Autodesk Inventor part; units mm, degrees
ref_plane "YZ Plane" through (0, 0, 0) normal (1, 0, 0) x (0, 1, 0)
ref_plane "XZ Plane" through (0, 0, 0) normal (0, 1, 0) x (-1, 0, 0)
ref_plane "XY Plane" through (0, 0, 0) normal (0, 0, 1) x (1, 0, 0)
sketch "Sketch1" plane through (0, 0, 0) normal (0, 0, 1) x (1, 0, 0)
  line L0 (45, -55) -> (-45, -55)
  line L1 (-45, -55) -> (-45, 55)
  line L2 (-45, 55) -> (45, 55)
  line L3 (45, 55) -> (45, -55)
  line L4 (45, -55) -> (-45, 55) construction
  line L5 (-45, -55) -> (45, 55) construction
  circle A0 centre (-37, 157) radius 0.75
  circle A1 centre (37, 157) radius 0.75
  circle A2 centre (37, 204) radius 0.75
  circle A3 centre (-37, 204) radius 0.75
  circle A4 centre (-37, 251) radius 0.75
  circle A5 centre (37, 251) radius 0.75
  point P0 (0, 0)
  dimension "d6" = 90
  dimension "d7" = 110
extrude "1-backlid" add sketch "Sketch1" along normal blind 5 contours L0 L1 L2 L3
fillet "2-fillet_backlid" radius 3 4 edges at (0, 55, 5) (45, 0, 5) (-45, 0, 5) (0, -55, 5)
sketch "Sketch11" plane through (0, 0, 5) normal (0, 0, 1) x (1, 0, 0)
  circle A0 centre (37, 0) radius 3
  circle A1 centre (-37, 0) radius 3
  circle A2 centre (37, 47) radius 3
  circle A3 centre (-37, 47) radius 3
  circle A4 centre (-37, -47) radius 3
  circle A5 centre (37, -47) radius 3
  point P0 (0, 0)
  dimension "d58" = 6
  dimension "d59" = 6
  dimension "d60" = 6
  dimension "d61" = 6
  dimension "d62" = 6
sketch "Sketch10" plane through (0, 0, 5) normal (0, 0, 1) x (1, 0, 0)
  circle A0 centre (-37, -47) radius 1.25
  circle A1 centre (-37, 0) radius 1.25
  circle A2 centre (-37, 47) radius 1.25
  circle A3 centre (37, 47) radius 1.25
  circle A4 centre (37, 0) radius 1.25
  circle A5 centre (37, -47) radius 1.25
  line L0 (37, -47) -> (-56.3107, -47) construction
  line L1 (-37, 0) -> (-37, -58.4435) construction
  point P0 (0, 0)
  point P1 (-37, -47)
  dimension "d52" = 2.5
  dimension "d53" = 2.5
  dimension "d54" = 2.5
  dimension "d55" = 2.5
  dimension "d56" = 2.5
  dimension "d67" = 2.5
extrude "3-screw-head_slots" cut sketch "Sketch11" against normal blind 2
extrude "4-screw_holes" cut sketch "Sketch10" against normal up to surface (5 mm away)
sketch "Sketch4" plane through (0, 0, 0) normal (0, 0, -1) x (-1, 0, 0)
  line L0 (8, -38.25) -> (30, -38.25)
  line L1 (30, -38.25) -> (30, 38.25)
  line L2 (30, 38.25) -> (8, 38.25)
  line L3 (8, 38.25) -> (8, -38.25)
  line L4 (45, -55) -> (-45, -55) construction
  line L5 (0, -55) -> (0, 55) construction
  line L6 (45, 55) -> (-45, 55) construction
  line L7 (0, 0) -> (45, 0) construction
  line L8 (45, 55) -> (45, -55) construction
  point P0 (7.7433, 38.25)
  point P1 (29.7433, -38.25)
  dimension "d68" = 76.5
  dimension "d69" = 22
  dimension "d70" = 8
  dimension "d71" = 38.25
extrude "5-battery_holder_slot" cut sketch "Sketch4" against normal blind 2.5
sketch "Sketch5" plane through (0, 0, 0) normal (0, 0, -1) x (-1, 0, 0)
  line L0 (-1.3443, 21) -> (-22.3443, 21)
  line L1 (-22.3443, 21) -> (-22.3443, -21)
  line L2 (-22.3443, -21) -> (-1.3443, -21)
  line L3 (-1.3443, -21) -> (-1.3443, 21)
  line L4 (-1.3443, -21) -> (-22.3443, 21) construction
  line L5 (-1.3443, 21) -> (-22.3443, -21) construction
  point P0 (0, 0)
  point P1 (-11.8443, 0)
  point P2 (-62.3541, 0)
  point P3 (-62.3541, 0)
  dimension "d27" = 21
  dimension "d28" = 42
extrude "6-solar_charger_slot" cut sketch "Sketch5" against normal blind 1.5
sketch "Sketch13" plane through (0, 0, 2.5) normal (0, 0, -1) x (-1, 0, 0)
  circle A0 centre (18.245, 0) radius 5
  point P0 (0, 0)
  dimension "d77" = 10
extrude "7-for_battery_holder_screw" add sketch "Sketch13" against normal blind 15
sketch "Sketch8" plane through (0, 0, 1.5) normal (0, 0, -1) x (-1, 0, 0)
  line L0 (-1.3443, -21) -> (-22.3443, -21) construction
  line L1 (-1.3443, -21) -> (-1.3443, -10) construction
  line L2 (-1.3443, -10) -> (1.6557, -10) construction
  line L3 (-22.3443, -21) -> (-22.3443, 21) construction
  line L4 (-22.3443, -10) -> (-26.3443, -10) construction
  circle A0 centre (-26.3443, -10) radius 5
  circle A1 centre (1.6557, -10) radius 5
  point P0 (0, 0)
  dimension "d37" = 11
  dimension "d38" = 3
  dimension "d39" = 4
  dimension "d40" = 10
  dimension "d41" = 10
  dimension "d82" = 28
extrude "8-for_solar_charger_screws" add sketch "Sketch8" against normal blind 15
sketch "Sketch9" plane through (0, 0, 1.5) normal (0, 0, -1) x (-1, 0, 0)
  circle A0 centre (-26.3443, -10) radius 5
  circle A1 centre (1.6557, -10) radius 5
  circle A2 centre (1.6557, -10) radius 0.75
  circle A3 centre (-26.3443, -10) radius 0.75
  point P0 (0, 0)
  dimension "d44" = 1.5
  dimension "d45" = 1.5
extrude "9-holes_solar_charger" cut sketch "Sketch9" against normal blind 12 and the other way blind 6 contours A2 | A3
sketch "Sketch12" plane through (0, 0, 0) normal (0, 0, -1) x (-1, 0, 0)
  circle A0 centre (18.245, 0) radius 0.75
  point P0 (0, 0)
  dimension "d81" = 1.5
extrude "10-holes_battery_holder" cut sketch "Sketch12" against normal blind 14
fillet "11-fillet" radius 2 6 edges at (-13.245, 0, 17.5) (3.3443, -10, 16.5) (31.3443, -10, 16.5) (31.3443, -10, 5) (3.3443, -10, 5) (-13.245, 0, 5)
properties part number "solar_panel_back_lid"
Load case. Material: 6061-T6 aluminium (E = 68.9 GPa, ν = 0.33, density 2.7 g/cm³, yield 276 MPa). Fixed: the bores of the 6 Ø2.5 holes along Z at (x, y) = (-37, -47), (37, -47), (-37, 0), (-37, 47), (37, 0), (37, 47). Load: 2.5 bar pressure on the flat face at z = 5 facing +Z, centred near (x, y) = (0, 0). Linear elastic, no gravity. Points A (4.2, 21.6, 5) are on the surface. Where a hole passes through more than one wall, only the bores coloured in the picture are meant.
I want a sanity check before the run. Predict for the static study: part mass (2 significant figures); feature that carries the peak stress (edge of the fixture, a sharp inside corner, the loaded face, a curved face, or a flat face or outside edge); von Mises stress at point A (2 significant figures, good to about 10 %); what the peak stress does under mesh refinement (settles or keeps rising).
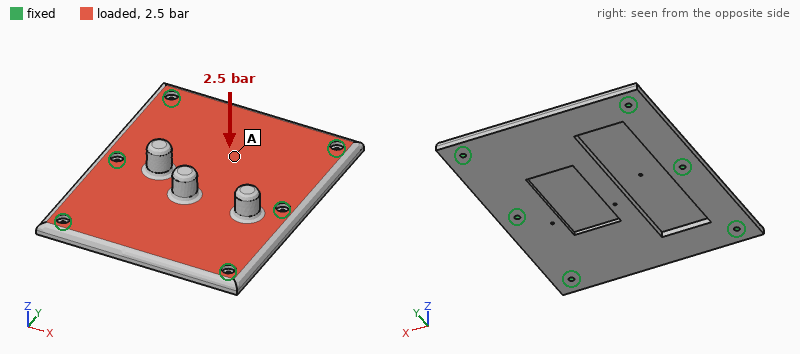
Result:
120 g
edge of the fixture
20 MPa
keeps rising
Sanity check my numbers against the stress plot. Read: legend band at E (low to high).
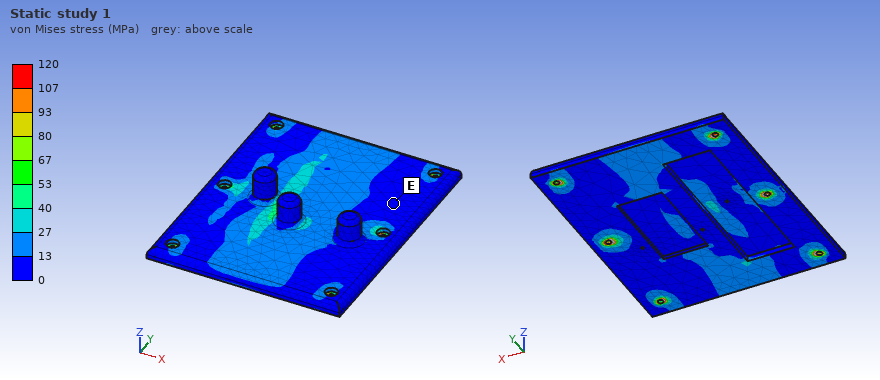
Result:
0 to 13 MPa
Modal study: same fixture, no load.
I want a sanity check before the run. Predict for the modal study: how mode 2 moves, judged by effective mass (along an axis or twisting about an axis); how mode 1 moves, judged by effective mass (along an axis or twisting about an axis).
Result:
twisting about X
along Z
